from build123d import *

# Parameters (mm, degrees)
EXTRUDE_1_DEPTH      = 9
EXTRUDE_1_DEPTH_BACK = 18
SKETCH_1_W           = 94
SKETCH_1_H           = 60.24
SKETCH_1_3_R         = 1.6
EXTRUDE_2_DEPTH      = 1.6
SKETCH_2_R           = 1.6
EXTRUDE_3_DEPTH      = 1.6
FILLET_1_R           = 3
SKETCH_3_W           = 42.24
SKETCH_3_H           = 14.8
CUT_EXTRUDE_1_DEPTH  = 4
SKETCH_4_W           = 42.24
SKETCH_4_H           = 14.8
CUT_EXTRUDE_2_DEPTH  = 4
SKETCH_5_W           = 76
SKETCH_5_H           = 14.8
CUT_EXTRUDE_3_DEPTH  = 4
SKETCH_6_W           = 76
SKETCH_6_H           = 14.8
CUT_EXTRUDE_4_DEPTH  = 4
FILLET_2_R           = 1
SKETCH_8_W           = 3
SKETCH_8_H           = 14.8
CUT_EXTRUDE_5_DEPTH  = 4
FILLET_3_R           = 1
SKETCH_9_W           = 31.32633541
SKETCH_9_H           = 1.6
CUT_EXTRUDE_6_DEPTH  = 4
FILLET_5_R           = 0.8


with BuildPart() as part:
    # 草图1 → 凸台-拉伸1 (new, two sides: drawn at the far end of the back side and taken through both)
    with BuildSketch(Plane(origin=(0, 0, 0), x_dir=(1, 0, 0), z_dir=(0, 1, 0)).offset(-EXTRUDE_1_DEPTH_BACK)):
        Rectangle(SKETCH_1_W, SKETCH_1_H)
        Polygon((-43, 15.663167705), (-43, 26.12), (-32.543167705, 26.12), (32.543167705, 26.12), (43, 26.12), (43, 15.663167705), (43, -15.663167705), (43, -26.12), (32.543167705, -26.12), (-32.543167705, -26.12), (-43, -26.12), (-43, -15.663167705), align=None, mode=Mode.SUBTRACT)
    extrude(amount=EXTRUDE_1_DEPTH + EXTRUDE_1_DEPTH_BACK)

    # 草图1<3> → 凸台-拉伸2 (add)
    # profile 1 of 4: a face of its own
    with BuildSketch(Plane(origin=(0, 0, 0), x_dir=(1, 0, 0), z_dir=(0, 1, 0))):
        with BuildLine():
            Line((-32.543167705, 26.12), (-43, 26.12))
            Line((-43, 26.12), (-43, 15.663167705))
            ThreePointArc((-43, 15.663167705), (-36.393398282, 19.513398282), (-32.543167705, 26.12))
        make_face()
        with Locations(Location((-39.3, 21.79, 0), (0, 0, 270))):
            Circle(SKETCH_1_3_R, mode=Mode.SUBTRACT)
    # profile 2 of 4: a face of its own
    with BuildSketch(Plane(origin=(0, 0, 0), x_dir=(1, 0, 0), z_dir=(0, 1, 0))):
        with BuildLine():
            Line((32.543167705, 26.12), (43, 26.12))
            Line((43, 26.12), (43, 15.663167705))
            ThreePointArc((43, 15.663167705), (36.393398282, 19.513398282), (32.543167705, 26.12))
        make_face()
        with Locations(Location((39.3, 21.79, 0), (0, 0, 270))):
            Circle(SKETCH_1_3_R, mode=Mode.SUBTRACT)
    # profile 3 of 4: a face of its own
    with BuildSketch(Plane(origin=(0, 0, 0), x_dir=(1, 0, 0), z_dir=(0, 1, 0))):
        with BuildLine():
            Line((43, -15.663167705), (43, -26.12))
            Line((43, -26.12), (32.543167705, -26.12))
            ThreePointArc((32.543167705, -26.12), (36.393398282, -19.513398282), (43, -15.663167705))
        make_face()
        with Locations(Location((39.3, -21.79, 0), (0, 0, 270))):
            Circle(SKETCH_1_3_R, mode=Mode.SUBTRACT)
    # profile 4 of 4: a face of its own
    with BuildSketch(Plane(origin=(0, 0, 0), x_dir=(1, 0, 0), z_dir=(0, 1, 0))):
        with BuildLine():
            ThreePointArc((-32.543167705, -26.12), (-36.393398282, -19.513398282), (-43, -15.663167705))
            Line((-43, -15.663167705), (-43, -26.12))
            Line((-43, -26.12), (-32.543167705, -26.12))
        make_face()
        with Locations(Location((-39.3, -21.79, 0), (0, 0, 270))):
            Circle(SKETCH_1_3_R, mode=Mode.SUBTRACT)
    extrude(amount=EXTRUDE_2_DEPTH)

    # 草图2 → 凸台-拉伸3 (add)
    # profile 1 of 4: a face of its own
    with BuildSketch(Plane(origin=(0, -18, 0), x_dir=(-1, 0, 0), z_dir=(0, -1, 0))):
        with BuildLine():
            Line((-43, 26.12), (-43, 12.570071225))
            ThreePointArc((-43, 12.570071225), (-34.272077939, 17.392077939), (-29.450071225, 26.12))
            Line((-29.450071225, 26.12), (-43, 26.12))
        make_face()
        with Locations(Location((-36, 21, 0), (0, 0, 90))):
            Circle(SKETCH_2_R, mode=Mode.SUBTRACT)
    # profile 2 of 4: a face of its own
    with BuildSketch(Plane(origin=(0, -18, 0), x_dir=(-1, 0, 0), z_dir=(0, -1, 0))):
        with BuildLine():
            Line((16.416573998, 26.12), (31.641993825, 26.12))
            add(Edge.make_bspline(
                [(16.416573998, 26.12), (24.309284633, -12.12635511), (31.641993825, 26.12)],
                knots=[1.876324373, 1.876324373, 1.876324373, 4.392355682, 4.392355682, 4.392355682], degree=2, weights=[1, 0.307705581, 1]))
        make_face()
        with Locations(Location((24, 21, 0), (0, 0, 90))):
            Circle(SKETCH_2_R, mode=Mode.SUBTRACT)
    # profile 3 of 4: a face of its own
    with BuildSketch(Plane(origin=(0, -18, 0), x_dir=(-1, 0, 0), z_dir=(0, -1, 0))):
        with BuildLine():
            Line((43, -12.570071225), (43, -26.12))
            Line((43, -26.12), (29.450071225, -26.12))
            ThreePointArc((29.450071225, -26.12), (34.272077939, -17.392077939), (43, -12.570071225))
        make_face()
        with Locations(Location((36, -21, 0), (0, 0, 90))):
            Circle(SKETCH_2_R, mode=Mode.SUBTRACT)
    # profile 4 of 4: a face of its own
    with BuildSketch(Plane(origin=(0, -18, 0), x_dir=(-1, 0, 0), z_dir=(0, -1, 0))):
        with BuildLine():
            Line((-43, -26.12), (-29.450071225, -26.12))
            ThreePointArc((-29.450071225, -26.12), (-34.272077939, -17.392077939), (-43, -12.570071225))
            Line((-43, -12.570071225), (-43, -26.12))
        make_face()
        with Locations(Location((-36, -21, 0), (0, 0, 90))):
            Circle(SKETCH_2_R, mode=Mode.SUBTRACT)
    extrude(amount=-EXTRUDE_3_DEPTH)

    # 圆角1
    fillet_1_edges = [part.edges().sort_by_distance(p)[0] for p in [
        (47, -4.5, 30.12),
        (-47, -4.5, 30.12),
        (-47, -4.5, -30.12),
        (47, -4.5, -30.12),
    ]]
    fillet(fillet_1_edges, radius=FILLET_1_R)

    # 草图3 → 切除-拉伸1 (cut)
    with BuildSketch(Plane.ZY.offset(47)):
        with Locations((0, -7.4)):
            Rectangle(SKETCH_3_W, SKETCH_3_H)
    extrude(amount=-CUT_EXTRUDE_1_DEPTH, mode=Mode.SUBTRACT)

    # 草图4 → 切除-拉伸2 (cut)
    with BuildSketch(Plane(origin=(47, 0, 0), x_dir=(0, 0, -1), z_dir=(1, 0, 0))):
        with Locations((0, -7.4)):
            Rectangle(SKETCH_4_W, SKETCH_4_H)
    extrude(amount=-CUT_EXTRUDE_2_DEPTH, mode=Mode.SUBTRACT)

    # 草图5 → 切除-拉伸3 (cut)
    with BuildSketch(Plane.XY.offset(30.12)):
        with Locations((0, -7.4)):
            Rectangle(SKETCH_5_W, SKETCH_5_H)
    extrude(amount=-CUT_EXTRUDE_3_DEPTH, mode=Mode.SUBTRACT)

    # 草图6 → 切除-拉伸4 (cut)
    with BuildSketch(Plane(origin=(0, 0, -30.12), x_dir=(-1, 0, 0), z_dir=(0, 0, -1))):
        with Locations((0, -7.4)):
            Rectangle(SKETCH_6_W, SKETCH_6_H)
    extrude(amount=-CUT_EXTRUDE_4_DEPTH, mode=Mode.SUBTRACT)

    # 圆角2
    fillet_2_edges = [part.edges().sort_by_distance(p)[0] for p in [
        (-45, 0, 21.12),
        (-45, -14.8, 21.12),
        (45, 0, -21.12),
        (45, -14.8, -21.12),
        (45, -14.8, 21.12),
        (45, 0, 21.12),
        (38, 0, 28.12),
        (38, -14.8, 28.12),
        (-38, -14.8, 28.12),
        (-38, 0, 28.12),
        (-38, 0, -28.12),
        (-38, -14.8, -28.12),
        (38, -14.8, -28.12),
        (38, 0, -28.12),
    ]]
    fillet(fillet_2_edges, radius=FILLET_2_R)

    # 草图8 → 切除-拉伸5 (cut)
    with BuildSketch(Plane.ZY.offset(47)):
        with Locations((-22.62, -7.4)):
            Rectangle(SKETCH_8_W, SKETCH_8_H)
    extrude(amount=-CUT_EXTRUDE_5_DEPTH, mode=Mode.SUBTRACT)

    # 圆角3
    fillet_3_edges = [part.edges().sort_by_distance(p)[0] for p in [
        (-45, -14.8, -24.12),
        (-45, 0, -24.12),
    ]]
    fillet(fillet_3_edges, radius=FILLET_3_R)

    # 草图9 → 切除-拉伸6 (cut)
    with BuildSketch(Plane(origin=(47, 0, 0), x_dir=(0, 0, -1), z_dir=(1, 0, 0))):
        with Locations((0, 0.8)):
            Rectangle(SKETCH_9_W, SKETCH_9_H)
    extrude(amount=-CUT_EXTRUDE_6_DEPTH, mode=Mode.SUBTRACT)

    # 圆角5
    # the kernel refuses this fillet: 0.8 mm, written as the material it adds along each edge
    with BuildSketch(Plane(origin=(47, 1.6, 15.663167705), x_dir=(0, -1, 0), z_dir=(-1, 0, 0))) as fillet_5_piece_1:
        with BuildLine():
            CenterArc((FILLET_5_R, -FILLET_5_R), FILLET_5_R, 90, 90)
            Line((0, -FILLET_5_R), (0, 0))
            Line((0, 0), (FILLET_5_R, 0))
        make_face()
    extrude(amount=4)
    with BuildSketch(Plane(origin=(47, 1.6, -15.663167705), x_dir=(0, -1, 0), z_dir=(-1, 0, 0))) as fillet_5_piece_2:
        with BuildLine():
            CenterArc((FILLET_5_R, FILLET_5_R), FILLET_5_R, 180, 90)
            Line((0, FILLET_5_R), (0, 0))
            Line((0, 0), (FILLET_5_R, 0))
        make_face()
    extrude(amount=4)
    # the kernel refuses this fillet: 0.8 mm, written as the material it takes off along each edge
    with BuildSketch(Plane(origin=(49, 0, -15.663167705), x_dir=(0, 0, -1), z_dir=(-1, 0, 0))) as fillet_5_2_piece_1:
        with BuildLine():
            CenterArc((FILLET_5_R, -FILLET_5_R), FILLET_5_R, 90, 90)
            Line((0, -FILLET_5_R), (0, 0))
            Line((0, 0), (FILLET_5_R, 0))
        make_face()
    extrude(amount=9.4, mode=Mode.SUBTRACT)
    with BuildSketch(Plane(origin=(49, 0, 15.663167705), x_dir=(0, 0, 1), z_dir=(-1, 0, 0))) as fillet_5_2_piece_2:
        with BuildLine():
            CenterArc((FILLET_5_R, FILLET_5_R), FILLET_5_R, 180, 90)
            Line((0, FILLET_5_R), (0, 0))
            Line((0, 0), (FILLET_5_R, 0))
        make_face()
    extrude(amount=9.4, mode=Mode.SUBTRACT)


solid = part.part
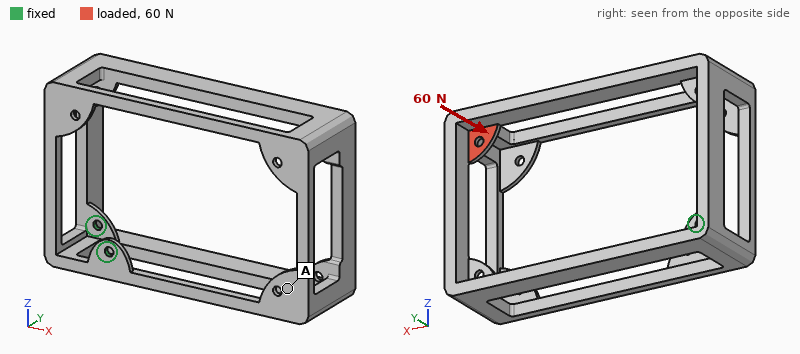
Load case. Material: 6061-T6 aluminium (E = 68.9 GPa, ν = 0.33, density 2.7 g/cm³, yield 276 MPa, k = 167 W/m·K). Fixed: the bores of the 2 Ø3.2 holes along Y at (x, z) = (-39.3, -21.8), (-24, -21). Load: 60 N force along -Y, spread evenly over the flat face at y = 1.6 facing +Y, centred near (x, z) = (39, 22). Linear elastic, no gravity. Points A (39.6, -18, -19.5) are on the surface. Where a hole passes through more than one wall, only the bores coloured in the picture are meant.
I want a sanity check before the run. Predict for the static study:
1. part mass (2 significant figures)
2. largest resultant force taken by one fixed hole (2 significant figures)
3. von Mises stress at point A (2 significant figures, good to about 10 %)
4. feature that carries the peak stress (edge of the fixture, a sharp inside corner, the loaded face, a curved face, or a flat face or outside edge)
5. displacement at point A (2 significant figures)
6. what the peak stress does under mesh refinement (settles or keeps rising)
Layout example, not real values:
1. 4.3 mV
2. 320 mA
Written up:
1. 49 g
2. 280 N
3. 11 MPa
4. edge of the fixture
5. 0.33 mm
6. keeps rising
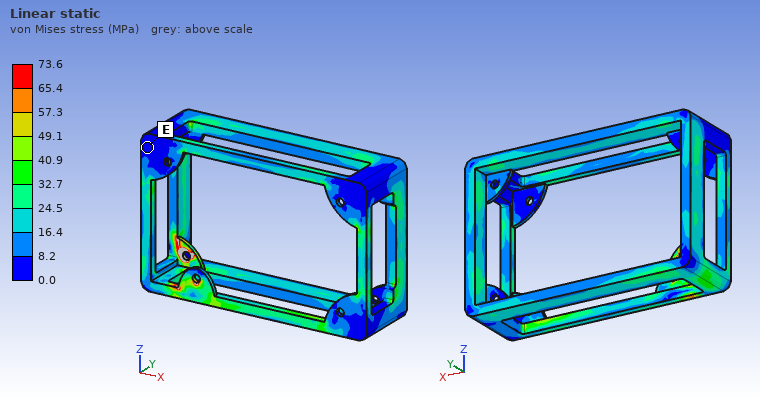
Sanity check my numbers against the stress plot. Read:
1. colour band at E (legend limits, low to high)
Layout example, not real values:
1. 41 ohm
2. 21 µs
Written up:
1. 0.0 to 8.2 MPa
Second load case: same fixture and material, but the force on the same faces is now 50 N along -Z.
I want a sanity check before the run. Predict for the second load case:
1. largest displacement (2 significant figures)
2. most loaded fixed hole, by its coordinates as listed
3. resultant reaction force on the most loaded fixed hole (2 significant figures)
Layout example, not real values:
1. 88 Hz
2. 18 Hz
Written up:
1. 0.87 mm
2. (-39.3, -21.8)
3. 35 N
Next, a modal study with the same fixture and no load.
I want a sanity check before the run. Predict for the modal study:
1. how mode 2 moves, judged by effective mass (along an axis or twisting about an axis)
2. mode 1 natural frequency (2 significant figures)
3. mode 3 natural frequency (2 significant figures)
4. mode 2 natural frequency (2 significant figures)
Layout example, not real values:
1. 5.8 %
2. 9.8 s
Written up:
1. along Y
2. 250 Hz
3. 740 Hz
4. 360 Hz
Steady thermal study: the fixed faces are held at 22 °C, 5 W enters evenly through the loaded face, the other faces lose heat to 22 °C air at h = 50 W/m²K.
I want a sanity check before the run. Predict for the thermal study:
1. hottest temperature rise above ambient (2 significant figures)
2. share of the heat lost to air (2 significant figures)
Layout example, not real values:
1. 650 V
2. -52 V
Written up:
1. 21 K
2. 83 %
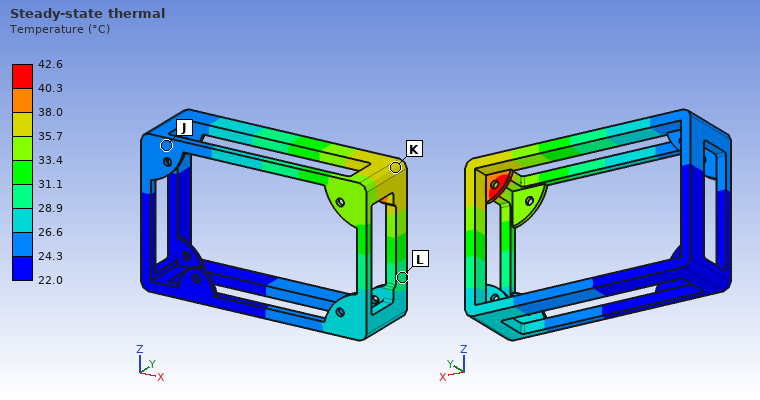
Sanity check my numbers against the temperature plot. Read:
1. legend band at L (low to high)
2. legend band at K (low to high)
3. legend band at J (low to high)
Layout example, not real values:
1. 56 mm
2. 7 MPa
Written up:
1. 28.9 to 31.1 °C
2. 35.7 to 38.0 °C
3. 24.3 to 26.6 °C
